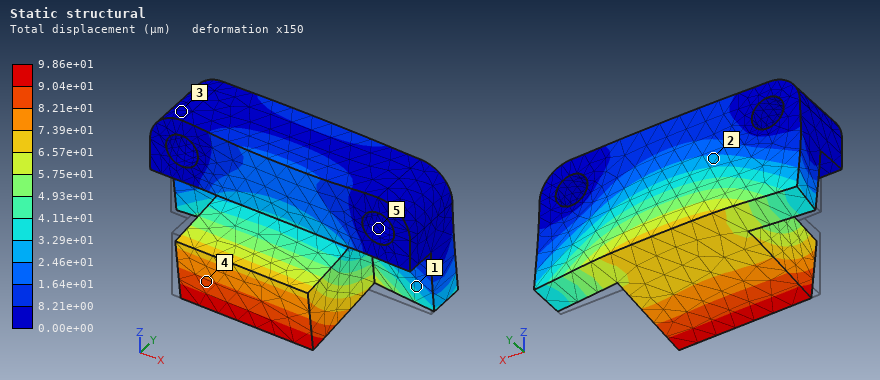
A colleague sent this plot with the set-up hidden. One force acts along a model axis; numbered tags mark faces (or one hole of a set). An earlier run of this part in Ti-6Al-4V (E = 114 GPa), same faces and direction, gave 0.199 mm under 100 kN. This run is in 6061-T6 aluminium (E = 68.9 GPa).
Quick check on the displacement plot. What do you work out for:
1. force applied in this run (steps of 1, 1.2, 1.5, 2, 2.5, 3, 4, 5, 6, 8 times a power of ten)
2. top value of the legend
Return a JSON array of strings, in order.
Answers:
["30 kN", "9.86e+01 µm"]
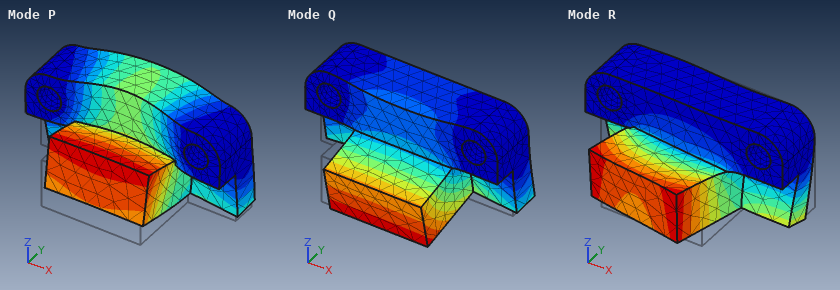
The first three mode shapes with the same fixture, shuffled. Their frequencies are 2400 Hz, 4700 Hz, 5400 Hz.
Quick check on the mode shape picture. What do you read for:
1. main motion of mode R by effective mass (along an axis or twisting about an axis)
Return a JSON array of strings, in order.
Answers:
["along X"]
